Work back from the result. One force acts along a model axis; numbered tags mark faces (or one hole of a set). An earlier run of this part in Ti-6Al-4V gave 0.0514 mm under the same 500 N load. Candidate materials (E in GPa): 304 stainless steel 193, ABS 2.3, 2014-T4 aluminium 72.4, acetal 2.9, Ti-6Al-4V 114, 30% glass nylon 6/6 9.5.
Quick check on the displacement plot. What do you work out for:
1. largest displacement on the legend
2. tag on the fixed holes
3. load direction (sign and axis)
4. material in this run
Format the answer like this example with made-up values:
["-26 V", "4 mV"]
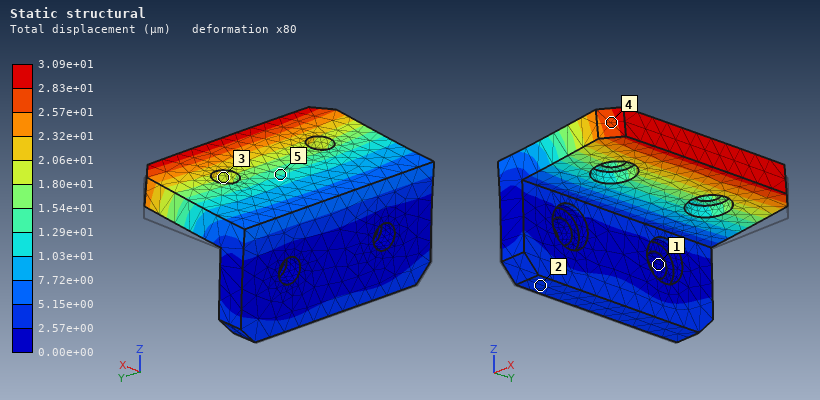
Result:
["3.09e+01 µm", "1", "+Z", "304 stainless steel"]
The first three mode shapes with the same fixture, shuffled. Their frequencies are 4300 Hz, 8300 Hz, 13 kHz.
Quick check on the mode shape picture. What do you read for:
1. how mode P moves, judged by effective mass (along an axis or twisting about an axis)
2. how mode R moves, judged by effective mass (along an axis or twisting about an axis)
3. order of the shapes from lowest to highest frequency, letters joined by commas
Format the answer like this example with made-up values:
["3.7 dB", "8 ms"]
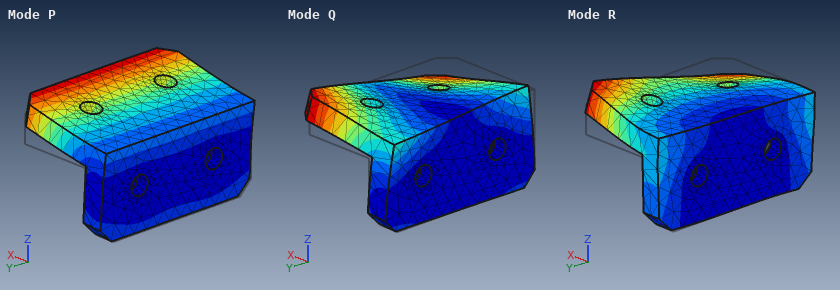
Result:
["along Z", "along Y", "P, Q, R"]
